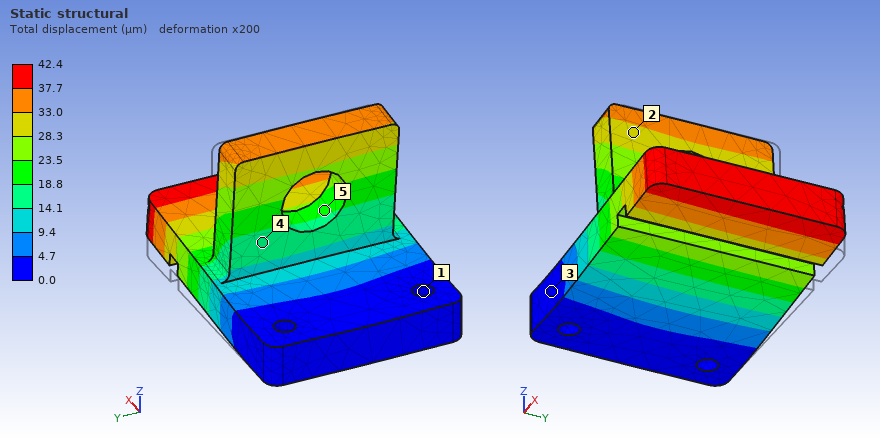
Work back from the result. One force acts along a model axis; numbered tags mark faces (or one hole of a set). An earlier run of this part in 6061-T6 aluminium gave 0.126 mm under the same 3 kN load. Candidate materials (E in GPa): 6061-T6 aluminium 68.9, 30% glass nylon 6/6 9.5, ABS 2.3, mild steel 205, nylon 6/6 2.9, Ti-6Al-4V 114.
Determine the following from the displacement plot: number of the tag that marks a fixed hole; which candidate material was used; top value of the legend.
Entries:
1
mild steel
42.4 µm
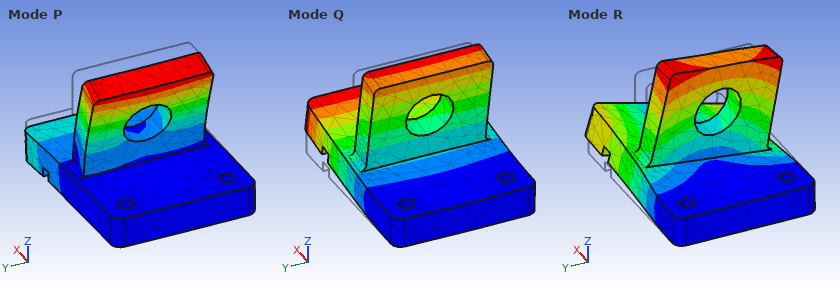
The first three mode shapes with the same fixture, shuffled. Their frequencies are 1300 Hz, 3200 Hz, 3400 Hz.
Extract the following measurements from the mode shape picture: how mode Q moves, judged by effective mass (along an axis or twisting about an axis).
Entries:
along Z
